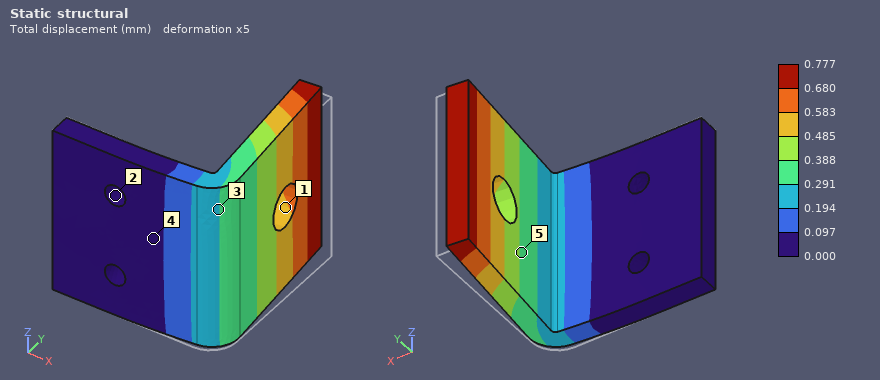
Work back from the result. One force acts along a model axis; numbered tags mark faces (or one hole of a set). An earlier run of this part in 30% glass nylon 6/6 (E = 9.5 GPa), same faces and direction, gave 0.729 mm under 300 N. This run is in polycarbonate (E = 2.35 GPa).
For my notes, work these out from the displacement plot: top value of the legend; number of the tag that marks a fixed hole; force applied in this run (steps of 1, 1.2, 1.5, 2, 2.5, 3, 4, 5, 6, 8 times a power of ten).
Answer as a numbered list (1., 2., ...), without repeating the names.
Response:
1. 0.777 mm
2. 2
3. 80 N
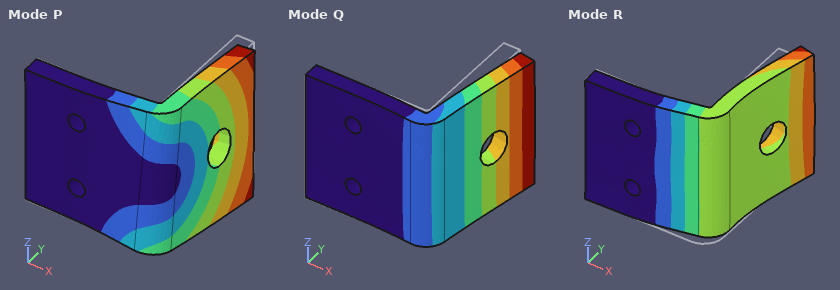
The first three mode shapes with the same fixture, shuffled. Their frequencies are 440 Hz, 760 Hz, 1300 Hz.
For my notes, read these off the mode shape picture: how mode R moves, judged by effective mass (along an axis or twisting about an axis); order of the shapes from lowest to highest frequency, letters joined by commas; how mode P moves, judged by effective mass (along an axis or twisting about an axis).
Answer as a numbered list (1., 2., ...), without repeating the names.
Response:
1. along Y
2. Q, P, R
3. along Z
